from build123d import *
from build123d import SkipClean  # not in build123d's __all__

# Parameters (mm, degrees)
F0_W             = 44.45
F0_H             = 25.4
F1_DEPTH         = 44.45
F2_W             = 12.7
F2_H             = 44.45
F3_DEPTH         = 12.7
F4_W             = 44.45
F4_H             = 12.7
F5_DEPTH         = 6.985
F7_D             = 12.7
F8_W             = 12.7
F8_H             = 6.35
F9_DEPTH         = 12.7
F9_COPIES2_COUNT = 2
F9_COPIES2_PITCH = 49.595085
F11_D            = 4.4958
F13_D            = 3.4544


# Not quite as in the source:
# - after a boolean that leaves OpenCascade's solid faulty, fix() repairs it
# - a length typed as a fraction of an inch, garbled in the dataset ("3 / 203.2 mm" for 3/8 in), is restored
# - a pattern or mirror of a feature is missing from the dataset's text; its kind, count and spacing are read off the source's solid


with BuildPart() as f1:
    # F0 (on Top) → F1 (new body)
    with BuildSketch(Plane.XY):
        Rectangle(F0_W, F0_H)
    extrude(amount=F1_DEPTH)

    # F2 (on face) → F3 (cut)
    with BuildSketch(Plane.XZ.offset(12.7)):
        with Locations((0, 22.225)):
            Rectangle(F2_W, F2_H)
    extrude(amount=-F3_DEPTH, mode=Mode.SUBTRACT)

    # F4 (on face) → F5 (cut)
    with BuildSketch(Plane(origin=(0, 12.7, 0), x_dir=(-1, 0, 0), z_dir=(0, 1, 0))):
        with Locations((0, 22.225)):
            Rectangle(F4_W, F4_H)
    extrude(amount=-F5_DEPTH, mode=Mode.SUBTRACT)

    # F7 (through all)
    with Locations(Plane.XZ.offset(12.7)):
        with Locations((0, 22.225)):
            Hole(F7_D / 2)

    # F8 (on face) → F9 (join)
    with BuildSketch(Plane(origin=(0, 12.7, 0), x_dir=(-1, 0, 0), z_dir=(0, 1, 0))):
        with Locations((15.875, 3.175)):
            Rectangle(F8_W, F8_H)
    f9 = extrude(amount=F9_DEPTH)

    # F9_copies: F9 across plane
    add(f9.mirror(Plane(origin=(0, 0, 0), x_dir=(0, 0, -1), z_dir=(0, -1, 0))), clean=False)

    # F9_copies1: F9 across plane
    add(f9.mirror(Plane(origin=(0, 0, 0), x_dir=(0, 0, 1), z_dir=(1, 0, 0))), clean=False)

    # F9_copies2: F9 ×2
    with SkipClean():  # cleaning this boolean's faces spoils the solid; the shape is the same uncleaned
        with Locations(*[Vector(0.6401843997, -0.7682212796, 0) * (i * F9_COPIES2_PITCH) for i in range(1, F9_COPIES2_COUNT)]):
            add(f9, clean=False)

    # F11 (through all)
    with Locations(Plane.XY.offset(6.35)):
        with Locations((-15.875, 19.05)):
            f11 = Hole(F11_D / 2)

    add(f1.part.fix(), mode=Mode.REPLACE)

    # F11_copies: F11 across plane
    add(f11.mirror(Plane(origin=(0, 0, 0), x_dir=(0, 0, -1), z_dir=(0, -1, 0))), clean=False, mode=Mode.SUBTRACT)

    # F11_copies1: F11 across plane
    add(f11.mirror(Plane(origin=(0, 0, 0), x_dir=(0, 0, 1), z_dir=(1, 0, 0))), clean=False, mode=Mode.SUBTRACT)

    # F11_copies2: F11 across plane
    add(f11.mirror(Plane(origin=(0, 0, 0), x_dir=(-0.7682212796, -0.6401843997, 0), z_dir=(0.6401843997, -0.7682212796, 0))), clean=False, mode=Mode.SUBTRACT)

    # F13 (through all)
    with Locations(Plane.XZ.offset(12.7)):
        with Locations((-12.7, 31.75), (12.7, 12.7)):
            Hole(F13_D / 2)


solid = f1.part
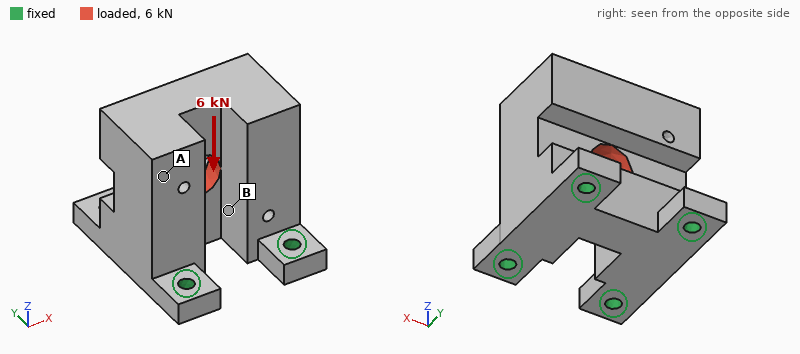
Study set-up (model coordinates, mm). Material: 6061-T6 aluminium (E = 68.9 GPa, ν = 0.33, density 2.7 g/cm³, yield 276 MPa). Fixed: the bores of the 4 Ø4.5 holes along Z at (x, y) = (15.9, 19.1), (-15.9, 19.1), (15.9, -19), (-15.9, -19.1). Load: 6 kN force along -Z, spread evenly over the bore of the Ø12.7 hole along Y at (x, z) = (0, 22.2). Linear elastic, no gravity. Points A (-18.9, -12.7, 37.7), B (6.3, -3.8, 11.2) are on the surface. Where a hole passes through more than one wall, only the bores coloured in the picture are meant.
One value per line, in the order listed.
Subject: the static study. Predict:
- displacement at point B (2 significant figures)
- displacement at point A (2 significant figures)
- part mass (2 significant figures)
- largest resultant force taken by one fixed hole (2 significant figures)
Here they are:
13 µm
14 µm
110 g
1.9 kN
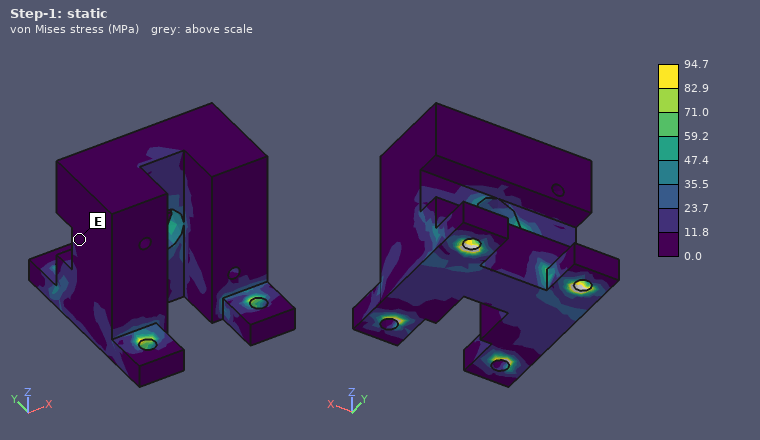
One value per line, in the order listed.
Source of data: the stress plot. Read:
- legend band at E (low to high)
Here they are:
0.0 to 11.8 MPa
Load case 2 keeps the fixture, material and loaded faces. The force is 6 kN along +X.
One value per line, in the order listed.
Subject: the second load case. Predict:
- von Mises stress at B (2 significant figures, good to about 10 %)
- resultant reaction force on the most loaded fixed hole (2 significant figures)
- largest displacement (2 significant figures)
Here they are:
25 MPa
2.8 kN
66 µm
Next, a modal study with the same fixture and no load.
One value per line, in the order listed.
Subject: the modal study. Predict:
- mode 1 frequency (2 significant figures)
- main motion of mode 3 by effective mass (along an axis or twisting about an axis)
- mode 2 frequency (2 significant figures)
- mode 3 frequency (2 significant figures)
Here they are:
5300 Hz
twisting about Z
5500 Hz
9100 Hz
